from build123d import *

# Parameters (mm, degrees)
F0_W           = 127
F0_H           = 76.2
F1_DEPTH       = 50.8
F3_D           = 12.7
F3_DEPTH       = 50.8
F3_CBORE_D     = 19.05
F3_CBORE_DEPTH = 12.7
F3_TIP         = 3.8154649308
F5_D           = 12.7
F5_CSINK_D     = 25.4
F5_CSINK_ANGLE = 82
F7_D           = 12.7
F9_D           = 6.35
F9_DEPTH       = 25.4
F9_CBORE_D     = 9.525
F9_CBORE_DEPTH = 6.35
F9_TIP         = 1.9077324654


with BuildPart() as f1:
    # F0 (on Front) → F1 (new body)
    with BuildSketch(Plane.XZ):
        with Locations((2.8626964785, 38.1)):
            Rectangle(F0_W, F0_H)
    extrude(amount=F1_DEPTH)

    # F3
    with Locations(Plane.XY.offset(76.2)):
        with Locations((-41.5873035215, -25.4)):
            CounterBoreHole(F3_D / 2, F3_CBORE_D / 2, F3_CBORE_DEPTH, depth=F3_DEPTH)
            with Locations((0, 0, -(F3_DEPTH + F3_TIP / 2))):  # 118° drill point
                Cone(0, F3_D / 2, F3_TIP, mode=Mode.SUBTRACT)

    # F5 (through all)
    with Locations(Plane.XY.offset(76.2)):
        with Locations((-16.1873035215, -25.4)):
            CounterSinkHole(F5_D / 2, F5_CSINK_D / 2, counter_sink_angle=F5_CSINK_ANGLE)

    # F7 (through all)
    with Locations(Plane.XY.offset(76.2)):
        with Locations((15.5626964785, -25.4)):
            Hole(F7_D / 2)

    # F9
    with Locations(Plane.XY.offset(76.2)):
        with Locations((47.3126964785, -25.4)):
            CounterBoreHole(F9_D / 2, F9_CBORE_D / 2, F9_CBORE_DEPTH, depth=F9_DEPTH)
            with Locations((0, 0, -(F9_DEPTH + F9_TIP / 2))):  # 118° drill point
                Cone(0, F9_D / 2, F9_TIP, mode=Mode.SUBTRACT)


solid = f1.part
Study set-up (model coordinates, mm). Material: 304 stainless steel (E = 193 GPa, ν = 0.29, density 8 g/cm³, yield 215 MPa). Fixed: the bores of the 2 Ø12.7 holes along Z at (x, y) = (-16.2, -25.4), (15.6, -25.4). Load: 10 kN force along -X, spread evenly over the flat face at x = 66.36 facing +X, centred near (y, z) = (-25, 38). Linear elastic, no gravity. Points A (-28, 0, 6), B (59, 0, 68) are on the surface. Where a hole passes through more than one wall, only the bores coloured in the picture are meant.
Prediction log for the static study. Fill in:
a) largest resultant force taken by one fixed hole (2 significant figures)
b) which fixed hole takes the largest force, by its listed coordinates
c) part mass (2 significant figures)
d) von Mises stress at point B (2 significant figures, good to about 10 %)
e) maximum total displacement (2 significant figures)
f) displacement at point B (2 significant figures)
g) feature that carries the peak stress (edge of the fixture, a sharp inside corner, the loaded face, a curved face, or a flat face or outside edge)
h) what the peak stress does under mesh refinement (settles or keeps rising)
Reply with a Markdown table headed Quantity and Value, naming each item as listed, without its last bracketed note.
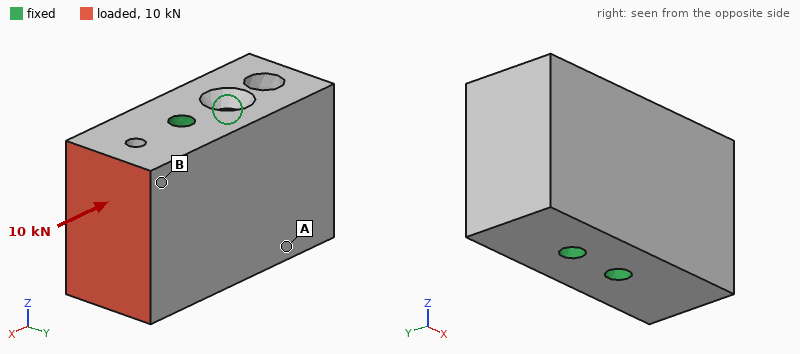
| Quantity | Value |
|---|---|
| largest resultant force taken by one fixed hole | 8.2 kN |
| which fixed hole takes the largest force, by its listed coordinates | (15.6, -25.4) |
| part mass | 3.7 kg |
| von Mises stress at point B | 2.5 MPa |
| maximum total displacement | 0.88 µm |
| displacement at point B | 0.69 µm |
| feature that carries the peak stress | a sharp inside corner |
| what the peak stress does under mesh refinement | keeps rising |
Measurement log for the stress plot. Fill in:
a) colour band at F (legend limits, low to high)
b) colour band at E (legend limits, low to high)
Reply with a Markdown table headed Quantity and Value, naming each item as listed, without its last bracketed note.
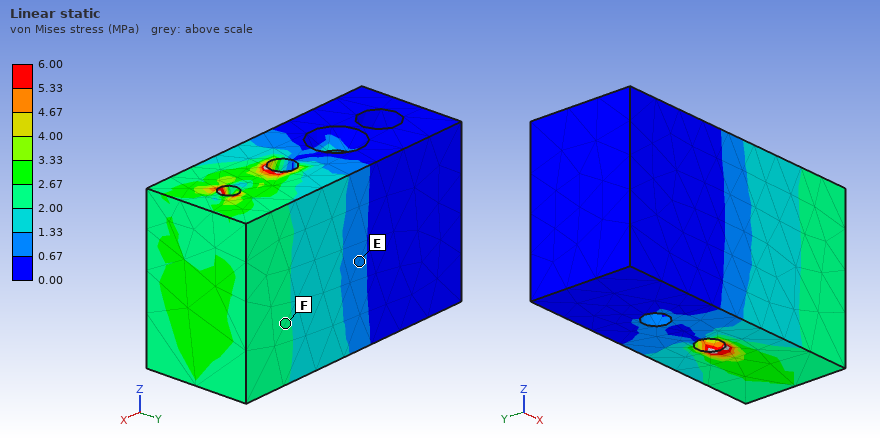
| Quantity | Value |
|---|---|
| colour band at F | 2.00 to 2.67 MPa |
| colour band at E | 0.67 to 1.33 MPa |
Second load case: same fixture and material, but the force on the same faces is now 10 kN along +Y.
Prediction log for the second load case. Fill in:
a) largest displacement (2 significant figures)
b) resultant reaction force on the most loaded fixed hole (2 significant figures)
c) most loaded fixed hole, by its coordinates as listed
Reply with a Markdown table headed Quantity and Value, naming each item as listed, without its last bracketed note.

| Quantity | Value |
|---|---|
| largest displacement | 8.6 µm |
| resultant reaction force on the most loaded fixed hole | 18 kN |
| most loaded fixed hole, by its coordinates as listed | (15.6, -25.4) |
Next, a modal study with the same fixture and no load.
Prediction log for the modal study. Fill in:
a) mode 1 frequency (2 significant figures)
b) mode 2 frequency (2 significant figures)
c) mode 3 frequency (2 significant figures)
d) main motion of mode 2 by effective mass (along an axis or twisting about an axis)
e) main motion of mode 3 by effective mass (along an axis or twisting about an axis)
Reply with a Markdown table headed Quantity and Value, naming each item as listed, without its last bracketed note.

| Quantity | Value |
|---|---|
| mode 1 frequency | 7600 Hz |
| mode 2 frequency | 9600 Hz |
| mode 3 frequency | 11 kHz |
| main motion of mode 2 by effective mass | along Y |
| main motion of mode 3 by effective mass | along Z |
